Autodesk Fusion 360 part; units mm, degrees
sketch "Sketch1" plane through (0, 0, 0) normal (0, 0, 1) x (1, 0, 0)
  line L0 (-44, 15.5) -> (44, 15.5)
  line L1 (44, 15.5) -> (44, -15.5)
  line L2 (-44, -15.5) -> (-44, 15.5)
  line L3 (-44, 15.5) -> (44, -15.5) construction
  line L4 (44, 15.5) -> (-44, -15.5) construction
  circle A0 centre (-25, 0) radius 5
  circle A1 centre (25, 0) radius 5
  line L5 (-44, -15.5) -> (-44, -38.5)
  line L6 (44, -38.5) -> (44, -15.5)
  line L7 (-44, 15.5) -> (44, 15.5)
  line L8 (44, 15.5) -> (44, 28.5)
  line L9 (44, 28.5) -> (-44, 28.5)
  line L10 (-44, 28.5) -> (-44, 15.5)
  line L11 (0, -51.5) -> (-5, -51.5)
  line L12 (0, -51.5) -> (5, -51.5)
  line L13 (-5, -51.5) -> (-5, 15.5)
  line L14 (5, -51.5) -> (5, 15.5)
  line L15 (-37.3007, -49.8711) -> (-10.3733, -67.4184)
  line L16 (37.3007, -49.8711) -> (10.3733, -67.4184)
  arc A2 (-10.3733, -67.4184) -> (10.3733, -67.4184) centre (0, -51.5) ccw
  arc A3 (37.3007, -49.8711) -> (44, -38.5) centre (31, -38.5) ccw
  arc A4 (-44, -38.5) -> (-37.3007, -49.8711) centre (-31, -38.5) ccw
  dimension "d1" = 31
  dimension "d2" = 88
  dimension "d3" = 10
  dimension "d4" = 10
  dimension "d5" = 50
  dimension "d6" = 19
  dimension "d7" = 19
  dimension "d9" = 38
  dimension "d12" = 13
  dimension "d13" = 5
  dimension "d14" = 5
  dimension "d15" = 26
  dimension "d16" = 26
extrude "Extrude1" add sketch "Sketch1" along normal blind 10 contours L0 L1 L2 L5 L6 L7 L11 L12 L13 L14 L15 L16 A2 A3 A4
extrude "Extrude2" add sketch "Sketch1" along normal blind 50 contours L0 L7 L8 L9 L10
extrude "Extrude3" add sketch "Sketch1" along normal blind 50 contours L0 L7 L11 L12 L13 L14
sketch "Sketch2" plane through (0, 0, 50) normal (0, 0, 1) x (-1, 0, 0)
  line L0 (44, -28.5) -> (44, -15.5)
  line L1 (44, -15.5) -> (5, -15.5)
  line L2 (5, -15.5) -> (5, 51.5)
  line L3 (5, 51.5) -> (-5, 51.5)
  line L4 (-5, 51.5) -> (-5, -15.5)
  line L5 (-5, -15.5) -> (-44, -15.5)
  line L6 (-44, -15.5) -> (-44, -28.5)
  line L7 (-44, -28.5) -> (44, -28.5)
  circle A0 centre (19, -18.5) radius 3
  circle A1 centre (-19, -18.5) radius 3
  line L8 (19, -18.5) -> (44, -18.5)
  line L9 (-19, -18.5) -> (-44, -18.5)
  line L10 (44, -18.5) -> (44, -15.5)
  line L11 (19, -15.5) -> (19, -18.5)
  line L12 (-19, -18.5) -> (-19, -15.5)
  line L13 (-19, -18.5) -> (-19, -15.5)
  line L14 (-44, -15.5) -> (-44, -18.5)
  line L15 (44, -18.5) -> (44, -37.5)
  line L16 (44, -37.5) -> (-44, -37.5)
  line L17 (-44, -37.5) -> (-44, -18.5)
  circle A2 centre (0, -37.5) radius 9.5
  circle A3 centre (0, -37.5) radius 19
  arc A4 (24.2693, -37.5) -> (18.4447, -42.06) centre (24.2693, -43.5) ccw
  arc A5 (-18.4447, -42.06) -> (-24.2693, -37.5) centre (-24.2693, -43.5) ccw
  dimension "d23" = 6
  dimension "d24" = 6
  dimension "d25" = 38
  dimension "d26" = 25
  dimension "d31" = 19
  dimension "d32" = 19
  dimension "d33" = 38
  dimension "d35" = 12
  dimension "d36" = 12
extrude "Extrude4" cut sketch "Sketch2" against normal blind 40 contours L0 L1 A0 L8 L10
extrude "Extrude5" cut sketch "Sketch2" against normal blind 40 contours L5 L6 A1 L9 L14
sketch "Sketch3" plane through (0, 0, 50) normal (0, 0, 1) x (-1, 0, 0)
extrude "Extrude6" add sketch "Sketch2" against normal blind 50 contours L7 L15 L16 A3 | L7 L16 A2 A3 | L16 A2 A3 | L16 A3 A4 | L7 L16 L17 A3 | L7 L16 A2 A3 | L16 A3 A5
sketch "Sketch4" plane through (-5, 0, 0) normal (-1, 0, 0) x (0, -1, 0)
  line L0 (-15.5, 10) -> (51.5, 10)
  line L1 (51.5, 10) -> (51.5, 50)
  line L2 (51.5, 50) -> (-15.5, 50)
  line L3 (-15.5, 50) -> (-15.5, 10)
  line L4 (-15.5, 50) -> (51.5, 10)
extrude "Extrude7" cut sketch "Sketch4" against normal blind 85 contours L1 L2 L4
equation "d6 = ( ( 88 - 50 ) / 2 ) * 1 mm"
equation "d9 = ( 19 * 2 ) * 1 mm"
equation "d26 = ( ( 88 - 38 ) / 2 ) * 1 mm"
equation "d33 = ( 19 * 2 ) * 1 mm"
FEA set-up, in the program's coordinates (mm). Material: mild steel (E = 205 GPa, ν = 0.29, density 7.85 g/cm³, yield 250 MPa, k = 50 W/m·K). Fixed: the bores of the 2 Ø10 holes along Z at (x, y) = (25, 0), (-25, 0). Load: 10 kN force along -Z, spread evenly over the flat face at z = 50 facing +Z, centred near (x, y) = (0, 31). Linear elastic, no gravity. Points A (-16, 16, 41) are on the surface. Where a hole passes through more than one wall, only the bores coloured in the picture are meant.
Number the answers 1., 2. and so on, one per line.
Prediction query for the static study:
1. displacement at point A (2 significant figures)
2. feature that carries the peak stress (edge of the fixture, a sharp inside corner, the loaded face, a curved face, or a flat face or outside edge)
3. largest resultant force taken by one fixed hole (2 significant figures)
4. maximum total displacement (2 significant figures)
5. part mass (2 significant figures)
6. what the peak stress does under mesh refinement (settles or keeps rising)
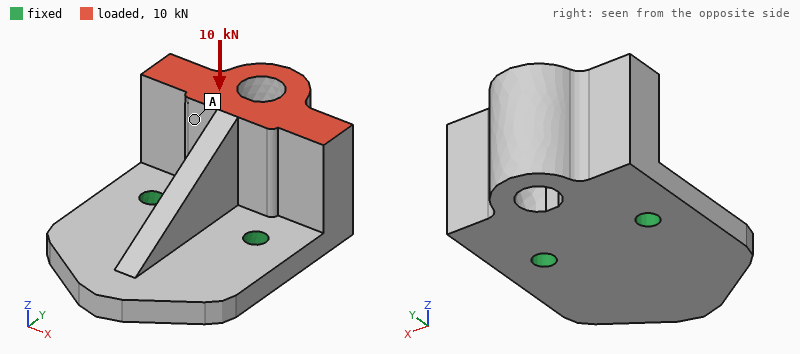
1. 51 µm
2. edge of the fixture
3. 5.1 kN
4. 96 µm
5. 1.4 kg
6. keeps rising
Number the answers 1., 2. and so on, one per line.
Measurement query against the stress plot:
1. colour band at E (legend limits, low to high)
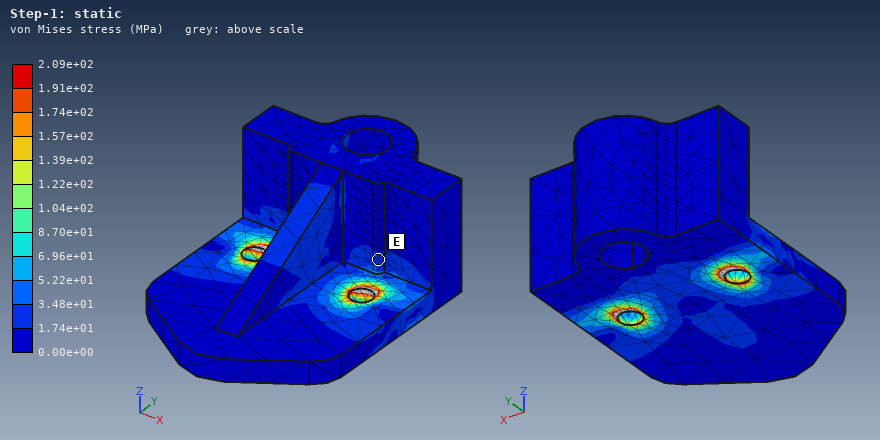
1. 1.74e+01 to 3.48e+01 MPa
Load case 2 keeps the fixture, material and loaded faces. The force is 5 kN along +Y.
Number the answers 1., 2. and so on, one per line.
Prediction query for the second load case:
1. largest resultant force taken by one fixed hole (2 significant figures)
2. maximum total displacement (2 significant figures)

1. 2.5 kN
2. 83 µm
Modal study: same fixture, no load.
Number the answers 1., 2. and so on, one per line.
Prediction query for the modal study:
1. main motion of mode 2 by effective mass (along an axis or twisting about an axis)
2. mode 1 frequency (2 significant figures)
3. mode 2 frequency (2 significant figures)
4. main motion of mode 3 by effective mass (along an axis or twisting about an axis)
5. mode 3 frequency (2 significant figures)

1. along X
2. 1800 Hz
3. 3900 Hz
4. along Z
5. 4200 Hz
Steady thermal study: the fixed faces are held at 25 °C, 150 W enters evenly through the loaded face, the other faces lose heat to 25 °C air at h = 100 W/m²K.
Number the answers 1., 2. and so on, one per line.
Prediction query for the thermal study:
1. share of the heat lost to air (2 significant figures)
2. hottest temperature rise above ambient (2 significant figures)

1. 60 %
2. 75 K
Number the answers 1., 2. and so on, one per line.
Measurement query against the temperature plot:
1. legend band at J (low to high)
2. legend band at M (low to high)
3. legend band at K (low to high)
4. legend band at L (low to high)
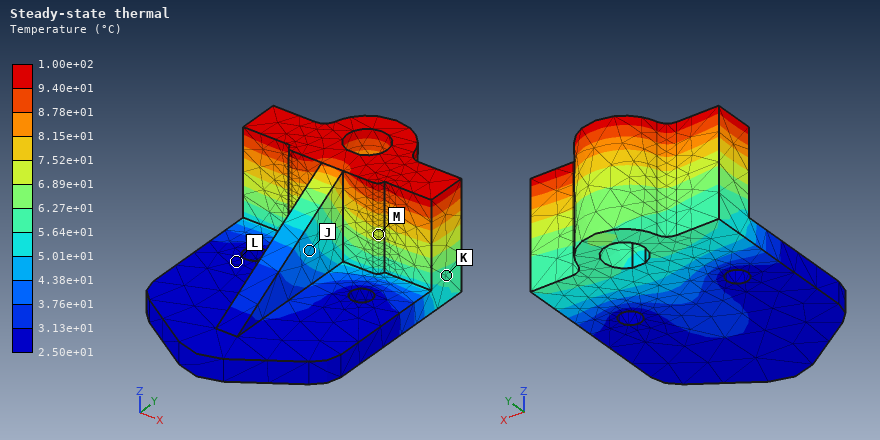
1. 4.38e+01 to 5.01e+01 °C
2. 6.89e+01 to 7.52e+01 °C
3. 5.64e+01 to 6.27e+01 °C
4. 2.50e+01 to 3.13e+01 °C
